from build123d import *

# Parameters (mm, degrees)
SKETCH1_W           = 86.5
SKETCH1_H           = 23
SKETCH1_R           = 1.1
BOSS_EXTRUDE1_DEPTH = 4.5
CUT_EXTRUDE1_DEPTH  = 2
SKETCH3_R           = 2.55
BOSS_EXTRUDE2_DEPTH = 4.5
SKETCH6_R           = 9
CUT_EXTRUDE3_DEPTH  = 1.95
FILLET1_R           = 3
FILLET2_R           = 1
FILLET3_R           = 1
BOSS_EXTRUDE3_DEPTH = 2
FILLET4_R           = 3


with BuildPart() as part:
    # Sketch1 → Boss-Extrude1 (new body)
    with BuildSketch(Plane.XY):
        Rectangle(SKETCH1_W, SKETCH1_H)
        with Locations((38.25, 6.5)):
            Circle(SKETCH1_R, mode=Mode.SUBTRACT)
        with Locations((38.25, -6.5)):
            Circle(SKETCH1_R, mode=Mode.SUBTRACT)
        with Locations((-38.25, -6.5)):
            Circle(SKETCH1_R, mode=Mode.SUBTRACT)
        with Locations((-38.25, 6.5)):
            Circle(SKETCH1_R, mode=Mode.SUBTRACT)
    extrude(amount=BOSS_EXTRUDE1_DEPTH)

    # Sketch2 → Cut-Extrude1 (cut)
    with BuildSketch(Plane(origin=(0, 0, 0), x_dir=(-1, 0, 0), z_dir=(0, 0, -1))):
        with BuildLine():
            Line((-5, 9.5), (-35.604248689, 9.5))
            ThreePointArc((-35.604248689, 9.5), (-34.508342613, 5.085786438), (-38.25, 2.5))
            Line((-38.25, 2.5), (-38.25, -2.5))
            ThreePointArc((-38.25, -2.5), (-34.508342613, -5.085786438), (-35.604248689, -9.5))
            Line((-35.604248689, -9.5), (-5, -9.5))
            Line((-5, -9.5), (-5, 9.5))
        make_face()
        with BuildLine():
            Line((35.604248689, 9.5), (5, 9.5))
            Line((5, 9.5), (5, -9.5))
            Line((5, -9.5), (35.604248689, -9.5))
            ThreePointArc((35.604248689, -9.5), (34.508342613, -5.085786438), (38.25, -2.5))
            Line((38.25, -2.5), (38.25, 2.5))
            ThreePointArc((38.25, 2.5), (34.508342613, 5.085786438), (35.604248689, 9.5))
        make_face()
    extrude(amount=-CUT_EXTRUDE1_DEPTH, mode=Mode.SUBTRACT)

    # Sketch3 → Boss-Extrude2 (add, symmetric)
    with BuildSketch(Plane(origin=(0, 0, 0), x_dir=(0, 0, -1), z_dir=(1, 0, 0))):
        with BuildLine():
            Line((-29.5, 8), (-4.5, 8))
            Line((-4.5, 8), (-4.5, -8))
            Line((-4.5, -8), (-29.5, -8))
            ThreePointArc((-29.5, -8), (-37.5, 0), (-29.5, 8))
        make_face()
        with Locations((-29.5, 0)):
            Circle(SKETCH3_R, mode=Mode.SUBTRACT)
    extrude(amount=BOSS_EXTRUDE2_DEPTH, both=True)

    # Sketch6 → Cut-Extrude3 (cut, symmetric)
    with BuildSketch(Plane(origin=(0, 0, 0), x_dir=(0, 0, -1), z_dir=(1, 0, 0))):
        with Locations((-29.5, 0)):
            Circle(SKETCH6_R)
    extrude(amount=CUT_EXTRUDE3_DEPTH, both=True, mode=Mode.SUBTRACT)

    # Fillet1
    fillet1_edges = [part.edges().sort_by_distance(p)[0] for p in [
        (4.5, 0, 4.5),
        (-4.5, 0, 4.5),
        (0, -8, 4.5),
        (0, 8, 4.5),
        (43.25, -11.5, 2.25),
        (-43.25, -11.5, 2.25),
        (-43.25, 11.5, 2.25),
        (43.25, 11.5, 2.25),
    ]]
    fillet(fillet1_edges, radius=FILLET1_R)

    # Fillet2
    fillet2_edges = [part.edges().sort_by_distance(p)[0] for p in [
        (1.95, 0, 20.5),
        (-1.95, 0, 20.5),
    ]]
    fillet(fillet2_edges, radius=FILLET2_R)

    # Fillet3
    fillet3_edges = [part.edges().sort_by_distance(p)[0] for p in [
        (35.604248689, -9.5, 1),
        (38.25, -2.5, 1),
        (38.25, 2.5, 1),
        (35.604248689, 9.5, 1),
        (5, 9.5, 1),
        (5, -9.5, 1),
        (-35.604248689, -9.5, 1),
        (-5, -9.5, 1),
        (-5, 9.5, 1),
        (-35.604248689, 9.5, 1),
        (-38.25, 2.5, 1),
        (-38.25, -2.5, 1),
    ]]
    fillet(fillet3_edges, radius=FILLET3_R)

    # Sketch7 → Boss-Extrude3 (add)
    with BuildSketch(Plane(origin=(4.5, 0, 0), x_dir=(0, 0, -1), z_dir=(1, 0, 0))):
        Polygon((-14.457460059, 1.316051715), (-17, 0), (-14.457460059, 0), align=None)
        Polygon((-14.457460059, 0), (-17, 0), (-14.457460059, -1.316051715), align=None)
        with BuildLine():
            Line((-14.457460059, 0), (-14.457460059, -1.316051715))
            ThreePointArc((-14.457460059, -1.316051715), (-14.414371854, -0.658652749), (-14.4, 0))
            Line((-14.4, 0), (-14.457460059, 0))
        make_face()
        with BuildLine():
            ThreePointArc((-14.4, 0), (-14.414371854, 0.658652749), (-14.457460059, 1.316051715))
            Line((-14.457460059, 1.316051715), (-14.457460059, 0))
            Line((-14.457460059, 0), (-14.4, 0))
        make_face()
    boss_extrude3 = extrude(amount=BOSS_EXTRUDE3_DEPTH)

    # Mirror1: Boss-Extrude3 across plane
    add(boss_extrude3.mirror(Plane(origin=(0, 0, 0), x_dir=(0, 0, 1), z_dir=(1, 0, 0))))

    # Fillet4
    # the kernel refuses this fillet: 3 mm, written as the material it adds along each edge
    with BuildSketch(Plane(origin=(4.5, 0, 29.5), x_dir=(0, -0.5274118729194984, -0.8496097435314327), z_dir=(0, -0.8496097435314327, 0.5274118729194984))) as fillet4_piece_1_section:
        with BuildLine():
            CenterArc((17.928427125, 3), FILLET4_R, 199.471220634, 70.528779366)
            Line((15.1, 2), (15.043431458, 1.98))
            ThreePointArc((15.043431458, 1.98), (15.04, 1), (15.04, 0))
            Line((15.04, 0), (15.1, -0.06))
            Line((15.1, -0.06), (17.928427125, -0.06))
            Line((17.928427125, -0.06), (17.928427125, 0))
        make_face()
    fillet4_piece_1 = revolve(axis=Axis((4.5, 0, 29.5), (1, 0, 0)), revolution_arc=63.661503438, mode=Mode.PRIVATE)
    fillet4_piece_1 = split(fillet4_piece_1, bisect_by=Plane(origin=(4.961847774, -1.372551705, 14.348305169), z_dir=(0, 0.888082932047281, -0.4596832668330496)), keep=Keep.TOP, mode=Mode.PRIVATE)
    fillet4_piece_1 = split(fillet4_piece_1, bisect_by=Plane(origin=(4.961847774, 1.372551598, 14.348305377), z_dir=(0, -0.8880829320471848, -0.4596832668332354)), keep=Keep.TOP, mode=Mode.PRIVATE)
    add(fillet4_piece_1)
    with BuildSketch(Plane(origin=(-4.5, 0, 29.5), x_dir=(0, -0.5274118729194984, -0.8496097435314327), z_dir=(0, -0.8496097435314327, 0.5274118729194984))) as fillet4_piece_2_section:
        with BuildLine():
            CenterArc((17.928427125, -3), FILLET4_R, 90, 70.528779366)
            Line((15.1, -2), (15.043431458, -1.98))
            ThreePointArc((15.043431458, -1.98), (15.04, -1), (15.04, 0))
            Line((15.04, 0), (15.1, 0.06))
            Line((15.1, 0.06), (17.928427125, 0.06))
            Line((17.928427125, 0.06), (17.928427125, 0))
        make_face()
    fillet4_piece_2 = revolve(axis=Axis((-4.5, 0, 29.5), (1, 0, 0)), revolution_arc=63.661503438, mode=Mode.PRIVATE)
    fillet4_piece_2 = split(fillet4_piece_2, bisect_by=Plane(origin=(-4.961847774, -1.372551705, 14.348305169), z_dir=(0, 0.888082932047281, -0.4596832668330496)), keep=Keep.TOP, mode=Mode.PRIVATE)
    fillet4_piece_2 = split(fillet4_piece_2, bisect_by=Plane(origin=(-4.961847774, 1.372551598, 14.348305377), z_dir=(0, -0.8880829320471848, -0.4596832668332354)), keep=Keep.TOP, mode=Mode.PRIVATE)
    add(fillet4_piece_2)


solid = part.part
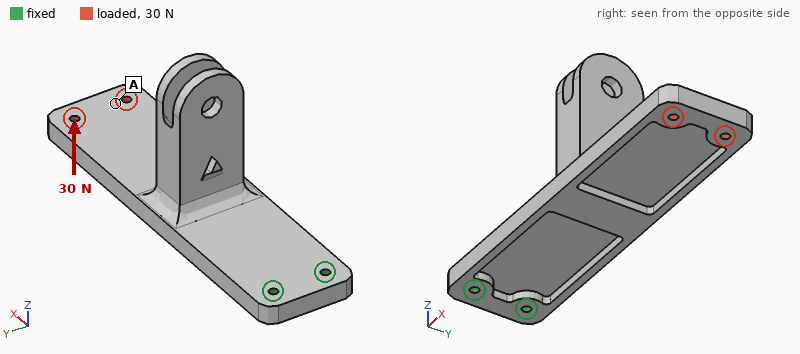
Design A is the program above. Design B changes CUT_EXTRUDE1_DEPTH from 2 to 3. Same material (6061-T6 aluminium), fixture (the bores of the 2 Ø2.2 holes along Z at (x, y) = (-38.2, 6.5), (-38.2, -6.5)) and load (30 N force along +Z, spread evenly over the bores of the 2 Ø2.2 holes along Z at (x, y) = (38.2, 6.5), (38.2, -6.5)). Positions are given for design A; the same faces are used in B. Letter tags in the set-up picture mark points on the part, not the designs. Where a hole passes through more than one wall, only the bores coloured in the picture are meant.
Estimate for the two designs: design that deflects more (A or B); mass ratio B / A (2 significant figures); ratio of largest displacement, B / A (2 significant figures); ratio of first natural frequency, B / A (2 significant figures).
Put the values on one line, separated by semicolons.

B; 0.89; 1.2; 0.98
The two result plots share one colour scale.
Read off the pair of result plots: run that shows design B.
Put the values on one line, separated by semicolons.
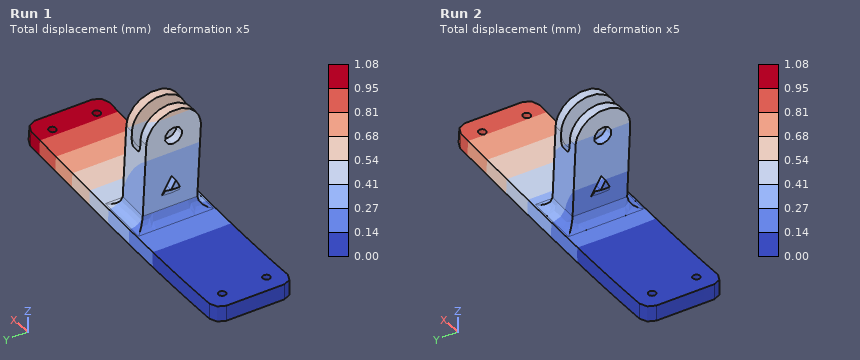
Run 1
